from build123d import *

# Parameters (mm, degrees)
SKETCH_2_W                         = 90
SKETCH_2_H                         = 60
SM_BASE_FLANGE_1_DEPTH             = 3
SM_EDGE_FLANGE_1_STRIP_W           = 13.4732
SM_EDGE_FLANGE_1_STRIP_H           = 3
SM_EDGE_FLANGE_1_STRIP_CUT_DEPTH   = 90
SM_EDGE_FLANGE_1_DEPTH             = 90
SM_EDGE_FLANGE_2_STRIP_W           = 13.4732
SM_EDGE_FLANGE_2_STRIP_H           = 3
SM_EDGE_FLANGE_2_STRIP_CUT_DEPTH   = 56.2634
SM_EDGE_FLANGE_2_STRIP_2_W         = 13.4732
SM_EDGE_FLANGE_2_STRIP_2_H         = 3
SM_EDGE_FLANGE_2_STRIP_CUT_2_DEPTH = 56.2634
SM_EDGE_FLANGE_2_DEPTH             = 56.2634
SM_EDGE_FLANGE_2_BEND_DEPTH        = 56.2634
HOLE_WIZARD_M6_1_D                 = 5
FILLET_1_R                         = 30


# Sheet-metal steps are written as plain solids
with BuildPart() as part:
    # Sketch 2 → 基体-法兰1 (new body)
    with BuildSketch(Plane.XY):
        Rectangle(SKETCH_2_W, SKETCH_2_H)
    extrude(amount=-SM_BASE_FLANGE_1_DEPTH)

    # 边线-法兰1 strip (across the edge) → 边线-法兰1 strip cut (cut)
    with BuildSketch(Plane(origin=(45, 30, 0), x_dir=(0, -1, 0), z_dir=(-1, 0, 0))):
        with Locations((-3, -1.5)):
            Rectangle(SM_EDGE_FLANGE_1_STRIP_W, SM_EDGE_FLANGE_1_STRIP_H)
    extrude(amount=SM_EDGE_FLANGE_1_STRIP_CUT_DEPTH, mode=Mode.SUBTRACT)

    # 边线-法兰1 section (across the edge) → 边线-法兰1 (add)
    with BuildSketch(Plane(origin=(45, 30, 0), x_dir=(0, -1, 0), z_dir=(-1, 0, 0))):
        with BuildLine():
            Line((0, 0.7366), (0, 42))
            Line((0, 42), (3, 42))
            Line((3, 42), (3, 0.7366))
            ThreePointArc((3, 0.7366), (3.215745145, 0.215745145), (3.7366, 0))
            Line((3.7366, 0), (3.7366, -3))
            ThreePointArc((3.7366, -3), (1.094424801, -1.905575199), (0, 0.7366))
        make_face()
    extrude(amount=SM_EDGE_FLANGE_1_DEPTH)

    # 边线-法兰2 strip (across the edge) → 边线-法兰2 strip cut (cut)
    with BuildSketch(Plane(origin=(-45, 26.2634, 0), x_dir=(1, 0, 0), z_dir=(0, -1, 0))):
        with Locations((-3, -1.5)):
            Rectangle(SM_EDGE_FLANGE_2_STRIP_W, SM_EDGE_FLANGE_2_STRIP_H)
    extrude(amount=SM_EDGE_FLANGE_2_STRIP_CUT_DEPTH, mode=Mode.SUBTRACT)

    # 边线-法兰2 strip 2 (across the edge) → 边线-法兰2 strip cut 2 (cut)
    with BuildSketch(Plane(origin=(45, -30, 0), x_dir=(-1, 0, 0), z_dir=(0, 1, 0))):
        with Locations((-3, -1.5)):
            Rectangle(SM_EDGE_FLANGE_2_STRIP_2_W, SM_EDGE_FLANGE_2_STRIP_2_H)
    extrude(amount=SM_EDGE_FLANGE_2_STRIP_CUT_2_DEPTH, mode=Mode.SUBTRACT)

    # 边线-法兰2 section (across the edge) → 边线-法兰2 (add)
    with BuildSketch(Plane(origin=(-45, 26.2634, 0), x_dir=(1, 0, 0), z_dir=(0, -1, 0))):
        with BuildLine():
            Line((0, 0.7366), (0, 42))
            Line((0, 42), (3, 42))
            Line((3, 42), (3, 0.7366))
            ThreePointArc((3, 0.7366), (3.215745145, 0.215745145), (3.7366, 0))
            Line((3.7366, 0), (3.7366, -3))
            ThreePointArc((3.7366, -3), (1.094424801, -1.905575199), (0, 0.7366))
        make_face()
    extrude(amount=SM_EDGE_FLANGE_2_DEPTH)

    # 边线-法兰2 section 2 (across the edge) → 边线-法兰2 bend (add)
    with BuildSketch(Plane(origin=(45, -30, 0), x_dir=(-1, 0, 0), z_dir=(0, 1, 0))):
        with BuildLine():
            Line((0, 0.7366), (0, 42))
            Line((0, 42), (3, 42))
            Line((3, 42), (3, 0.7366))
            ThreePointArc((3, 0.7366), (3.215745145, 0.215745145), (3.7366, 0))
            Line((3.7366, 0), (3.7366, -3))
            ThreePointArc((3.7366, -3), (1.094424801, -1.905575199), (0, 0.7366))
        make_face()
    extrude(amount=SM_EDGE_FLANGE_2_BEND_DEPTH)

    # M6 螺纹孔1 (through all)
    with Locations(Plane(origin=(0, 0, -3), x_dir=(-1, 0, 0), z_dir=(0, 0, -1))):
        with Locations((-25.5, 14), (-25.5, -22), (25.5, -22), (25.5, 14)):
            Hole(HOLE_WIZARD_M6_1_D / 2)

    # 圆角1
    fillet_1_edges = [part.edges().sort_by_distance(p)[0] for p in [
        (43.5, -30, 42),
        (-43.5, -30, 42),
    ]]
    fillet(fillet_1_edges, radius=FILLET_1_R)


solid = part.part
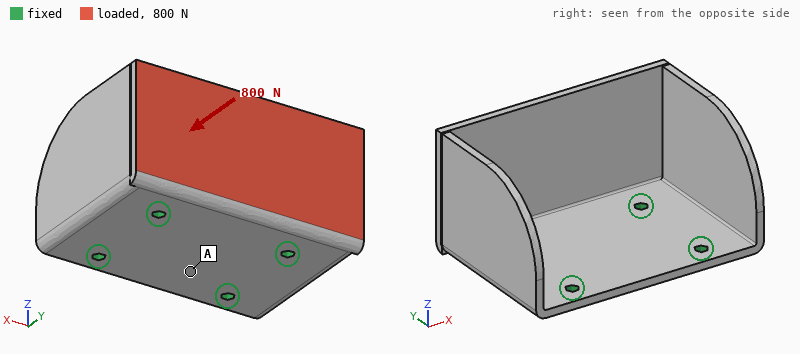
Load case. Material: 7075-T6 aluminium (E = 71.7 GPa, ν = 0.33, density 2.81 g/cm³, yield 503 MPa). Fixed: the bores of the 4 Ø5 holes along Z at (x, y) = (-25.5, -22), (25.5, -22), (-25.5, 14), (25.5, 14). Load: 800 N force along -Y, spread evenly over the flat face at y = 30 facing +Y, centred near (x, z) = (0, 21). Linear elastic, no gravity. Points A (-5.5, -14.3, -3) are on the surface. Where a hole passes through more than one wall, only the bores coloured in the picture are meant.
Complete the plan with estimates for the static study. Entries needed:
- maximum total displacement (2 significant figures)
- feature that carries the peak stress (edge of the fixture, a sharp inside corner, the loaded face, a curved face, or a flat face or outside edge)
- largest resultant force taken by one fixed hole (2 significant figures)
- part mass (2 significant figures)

1.1 mm
a curved face
330 N
110 g
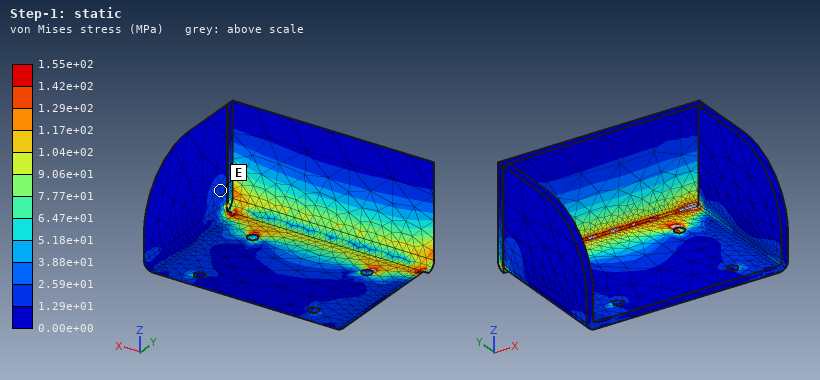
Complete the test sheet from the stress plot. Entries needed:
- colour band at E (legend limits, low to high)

1.29e+01 to 2.59e+01 MPa
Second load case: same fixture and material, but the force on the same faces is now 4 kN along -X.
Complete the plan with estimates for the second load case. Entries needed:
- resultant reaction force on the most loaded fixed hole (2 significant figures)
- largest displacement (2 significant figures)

2.8 kN
0.41 mm
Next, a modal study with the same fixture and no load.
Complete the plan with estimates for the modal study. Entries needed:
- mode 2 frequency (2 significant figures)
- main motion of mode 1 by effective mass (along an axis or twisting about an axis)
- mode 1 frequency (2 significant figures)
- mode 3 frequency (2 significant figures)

1000 Hz
along Y
920 Hz
1000 Hz
